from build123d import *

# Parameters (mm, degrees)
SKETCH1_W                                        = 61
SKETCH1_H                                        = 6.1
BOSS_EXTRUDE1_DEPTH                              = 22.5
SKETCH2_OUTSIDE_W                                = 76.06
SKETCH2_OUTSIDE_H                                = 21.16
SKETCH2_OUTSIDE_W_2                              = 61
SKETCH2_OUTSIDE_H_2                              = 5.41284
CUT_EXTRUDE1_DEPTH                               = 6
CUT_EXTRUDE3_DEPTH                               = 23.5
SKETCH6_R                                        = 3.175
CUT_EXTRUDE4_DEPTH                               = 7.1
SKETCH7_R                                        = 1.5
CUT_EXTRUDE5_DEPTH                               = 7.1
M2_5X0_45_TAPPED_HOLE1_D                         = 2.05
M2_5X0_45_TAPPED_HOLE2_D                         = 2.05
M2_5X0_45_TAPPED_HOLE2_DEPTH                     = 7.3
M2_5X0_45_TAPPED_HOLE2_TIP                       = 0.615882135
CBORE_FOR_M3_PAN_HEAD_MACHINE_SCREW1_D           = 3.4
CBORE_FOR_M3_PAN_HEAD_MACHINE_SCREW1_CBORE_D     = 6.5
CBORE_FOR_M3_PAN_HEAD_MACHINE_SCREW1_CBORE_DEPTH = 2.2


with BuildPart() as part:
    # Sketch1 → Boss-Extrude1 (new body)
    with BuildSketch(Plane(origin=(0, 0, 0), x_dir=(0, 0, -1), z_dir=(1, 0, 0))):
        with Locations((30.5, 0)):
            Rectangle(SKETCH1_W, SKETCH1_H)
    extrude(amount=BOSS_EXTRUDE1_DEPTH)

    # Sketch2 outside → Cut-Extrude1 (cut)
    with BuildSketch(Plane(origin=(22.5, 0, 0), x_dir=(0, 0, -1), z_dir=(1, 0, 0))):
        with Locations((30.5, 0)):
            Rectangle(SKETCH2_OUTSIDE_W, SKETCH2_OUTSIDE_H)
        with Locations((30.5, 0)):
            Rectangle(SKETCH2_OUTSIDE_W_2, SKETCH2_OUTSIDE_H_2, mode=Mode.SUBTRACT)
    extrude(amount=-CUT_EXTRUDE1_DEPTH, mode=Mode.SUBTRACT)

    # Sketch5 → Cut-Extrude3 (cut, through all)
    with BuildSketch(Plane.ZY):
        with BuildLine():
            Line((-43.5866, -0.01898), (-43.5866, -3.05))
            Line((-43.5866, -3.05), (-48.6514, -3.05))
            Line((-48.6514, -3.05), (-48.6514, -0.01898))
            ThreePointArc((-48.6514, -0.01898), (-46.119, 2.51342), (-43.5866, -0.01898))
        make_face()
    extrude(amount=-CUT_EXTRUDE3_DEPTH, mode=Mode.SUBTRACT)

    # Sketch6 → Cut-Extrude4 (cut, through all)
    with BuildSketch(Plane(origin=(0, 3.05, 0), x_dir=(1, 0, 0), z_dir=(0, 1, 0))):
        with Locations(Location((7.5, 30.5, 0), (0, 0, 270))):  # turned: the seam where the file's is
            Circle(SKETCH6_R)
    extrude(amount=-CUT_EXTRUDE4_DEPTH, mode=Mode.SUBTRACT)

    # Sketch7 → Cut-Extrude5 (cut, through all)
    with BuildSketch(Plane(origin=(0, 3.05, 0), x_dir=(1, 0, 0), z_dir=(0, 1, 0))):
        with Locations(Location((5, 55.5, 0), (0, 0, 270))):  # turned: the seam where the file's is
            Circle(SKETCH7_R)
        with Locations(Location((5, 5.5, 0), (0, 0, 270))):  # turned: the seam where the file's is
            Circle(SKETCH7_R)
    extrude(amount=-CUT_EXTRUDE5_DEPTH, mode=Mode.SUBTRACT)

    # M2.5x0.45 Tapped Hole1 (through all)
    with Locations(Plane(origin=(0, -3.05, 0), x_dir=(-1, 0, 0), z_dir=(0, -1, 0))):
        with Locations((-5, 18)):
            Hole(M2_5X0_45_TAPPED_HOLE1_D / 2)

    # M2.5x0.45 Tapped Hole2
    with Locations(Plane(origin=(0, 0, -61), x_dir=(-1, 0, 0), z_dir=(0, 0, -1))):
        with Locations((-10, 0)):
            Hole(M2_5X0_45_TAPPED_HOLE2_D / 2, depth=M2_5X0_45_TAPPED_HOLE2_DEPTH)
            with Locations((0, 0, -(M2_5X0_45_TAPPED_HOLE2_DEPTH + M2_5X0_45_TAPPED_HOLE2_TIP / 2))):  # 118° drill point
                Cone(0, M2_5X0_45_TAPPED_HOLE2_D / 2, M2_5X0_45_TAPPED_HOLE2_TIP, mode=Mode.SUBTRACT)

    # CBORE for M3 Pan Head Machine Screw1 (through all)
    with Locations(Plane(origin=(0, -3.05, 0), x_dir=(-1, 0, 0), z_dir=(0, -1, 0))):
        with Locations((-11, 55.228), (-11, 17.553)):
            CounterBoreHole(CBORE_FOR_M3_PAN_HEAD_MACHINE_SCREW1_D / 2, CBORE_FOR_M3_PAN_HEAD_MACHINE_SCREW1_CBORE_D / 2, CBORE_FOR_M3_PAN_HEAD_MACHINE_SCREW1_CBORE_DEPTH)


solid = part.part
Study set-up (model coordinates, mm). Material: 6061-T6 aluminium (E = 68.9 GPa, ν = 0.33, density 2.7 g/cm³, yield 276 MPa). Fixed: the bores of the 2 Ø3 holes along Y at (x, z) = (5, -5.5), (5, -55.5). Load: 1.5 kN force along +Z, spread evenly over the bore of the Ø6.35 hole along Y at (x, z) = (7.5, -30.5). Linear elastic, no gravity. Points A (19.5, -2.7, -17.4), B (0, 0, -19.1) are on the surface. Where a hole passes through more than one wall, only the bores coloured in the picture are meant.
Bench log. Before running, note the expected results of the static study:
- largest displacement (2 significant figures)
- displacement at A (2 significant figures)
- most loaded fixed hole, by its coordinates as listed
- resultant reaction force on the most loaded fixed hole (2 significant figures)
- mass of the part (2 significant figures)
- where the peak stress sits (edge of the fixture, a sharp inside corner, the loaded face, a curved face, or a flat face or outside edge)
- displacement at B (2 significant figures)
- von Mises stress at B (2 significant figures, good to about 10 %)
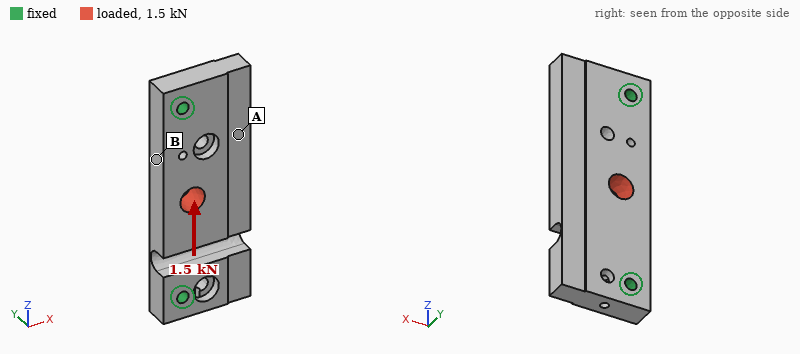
10 µm
6.0 µm
(5, -5.5)
1.2 kN
19 g
a curved face
3.5 µm
19 MPa
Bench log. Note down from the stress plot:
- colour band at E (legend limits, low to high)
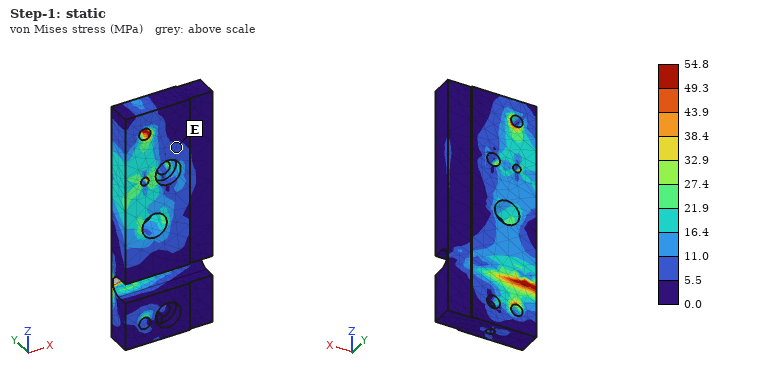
5.5 to 11.0 MPa
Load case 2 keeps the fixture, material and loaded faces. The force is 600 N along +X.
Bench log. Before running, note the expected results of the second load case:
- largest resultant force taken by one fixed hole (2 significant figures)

340 N
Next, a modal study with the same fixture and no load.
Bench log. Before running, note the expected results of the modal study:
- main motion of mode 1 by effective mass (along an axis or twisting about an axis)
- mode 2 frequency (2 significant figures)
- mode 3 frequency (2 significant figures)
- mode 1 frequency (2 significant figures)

along Y
9300 Hz
12 kHz
6200 Hz
